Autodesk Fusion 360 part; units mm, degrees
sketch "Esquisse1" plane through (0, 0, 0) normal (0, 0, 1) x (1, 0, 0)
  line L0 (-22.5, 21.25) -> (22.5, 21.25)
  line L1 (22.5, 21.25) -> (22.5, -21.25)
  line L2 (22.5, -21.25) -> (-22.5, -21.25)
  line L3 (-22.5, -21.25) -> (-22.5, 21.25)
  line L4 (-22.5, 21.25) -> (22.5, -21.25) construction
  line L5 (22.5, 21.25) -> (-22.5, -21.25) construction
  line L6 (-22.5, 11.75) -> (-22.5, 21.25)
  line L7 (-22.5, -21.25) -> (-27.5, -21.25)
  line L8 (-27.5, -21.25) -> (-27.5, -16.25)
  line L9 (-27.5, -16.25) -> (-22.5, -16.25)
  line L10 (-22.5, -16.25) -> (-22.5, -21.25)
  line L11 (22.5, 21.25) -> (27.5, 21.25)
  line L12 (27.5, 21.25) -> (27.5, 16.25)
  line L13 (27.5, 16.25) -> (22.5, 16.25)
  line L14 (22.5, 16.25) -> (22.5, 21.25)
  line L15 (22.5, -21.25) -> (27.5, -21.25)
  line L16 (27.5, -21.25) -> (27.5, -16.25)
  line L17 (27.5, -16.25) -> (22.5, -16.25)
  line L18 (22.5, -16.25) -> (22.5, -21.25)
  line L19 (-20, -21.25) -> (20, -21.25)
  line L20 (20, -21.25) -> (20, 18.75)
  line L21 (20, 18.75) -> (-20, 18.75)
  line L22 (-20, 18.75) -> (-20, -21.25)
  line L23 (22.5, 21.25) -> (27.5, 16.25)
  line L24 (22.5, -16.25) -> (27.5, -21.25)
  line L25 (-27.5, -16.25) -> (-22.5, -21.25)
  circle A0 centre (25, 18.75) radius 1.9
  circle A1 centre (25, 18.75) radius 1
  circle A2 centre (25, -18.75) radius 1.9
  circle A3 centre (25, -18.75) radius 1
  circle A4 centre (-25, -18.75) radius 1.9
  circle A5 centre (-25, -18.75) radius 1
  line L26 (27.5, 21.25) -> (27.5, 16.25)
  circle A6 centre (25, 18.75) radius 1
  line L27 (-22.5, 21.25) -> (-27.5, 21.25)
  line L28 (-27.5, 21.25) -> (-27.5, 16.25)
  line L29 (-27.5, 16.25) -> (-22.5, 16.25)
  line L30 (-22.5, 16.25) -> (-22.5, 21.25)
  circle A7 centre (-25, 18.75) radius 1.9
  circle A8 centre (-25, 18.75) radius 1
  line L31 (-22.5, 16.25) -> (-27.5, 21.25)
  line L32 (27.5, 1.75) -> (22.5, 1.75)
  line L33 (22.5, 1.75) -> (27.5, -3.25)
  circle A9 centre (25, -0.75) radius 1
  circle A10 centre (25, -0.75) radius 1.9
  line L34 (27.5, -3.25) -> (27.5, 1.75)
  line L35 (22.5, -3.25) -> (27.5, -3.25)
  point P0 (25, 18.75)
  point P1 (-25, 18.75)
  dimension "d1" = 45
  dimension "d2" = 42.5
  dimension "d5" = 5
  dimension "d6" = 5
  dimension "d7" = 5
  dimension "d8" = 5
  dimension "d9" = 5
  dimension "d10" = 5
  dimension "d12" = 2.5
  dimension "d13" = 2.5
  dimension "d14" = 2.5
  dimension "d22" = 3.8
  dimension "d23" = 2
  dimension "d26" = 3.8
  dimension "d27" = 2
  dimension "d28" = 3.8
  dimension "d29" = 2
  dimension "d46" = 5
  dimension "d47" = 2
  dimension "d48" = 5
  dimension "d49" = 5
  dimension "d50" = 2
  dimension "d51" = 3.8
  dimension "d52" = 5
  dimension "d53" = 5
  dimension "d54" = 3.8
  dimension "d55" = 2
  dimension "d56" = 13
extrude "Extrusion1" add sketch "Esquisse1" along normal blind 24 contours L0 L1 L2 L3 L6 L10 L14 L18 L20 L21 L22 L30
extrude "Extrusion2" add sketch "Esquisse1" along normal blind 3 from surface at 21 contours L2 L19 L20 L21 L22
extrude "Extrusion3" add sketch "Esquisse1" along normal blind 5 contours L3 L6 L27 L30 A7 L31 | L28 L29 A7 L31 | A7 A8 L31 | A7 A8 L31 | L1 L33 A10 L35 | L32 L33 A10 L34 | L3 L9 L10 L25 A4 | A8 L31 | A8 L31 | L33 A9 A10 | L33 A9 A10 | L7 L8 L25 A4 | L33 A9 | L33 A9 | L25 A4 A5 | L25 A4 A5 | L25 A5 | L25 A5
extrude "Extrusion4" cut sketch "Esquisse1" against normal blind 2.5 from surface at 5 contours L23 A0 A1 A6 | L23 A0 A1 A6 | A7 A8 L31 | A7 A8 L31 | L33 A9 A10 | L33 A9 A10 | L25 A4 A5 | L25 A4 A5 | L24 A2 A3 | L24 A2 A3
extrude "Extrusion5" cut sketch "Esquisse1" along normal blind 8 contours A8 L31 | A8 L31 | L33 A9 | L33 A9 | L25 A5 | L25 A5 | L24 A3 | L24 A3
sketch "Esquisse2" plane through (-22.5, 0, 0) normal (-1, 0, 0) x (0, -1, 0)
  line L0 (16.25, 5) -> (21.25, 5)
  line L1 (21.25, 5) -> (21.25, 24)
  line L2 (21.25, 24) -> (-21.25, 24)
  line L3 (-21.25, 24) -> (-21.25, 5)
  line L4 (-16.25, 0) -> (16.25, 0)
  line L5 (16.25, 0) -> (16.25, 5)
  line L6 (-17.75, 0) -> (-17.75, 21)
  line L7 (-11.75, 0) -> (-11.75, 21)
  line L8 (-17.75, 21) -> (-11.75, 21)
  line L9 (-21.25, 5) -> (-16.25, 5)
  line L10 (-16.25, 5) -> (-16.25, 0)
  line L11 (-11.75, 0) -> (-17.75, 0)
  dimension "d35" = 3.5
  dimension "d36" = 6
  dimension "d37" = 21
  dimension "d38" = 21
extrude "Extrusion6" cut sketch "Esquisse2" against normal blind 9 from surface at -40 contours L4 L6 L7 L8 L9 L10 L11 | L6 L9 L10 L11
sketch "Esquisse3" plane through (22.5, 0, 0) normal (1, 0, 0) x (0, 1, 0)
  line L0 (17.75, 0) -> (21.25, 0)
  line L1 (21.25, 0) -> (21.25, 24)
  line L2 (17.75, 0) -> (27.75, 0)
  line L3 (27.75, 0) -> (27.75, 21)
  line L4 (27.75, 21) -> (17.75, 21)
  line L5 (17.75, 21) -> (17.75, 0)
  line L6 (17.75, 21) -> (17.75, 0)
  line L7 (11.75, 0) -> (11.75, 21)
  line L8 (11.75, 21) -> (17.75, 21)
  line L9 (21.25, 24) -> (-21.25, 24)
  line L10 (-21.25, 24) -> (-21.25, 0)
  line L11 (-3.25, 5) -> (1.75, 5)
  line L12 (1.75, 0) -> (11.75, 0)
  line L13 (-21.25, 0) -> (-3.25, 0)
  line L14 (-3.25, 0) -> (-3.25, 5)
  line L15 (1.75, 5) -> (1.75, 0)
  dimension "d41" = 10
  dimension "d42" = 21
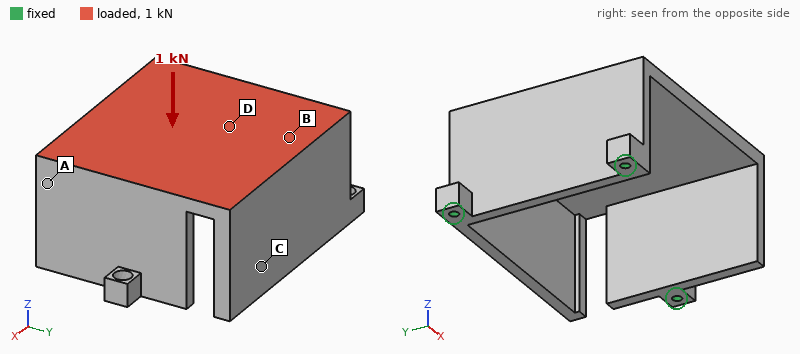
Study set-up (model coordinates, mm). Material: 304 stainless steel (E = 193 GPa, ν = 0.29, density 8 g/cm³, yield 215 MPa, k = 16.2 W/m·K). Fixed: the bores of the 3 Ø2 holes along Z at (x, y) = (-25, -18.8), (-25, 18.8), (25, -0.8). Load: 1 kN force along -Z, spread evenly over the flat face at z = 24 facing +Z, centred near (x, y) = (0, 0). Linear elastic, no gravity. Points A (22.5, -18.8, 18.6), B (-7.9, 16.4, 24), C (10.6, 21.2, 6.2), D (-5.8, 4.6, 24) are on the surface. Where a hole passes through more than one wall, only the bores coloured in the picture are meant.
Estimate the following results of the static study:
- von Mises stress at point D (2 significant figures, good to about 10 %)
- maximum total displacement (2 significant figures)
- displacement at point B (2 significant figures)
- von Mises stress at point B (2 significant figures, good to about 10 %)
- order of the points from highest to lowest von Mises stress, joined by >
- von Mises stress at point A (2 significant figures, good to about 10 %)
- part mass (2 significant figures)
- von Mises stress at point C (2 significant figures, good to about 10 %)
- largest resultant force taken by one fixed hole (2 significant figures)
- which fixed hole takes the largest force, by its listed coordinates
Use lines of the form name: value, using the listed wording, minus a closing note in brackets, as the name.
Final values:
von Mises stress at point D: 21 MPa
maximum total displacement: 25 µm
displacement at point B: 8.0 µm
von Mises stress at point B: 11 MPa
order of the points from highest to lowest von Mises stress, joined by >: A > D > B > C
von Mises stress at point A: 28 MPa
part mass: 98 g
von Mises stress at point C: 4.9 MPa
largest resultant force taken by one fixed hole: 510 N
which fixed hole takes the largest force, by its listed coordinates: (25, -0.8)
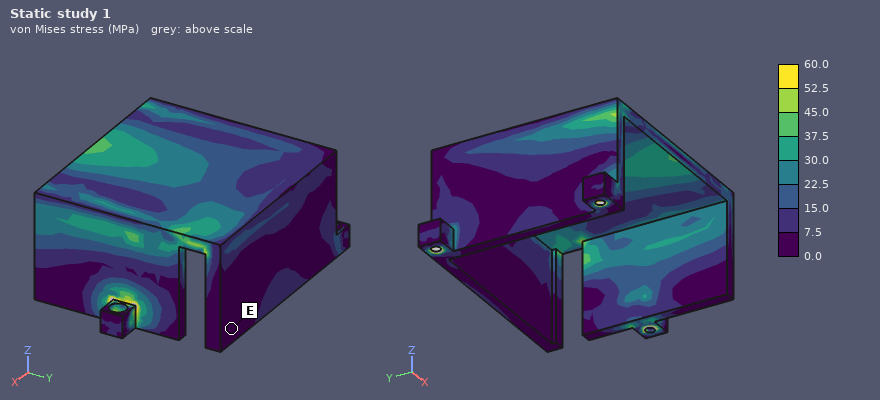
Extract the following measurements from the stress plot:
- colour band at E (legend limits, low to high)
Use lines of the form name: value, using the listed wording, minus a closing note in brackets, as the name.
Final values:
colour band at E: 0.0 to 7.5 MPa
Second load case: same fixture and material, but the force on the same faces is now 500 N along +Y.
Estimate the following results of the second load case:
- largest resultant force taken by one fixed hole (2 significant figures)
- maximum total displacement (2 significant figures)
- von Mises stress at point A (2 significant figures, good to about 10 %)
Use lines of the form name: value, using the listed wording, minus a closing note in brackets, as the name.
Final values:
largest resultant force taken by one fixed hole: 360 N
maximum total displacement: 40 µm
von Mises stress at point A: 20 MPa
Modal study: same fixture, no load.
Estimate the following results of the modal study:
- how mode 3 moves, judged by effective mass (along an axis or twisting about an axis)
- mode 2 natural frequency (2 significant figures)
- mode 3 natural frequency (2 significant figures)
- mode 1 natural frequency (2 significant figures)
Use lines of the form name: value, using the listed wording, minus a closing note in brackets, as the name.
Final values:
how mode 3 moves, judged by effective mass: along Z
mode 2 natural frequency: 3300 Hz
mode 3 natural frequency: 5500 Hz
mode 1 natural frequency: 2100 Hz
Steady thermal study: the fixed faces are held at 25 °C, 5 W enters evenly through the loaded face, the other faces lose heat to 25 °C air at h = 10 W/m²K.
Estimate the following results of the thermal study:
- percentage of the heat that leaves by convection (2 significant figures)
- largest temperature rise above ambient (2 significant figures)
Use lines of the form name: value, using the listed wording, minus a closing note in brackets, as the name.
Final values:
percentage of the heat that leaves by convection: 44 %
largest temperature rise above ambient: 43 K
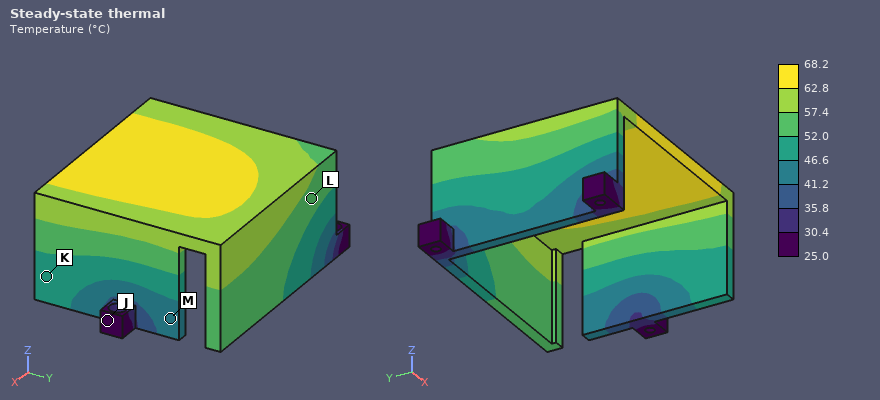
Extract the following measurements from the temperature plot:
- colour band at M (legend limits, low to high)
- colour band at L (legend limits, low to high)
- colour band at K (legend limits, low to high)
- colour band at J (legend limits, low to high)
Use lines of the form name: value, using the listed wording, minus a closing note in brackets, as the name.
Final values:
colour band at M: 41.2 to 46.6 °C
colour band at L: 52.0 to 57.4 °C
colour band at K: 46.6 to 52.0 °C
colour band at J: 25.0 to 30.4 °C
